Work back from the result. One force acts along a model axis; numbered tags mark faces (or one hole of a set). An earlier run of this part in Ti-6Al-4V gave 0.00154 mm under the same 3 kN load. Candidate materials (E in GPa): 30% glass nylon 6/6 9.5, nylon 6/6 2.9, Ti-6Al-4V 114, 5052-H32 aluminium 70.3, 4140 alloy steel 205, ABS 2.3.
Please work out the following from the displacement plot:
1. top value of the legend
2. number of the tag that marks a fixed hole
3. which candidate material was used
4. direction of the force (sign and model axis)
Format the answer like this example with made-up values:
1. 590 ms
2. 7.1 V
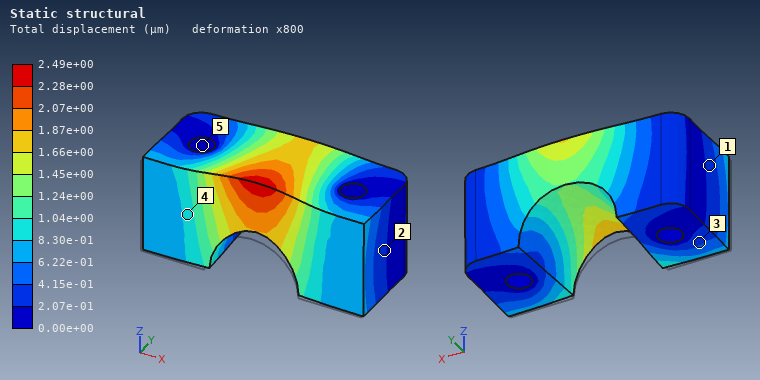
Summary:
1. 2.49e+00 µm
2. 5
3. 5052-H32 aluminium
4. +Y
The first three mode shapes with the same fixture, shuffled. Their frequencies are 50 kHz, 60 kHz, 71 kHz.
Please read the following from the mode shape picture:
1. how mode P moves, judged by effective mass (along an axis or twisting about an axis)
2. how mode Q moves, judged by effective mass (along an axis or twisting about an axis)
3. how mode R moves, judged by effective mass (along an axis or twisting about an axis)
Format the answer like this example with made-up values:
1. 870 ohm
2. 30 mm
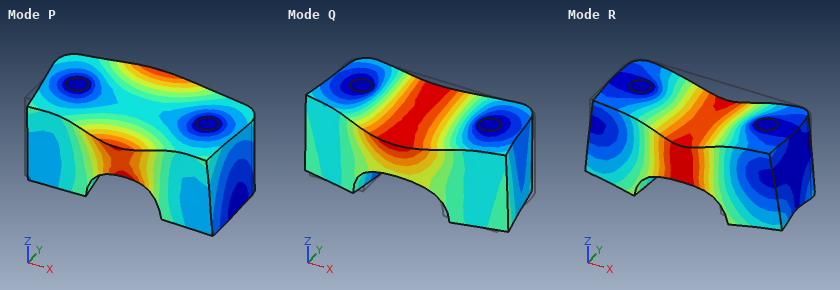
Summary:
1. twisting about X
2. along Y
3. along Z
